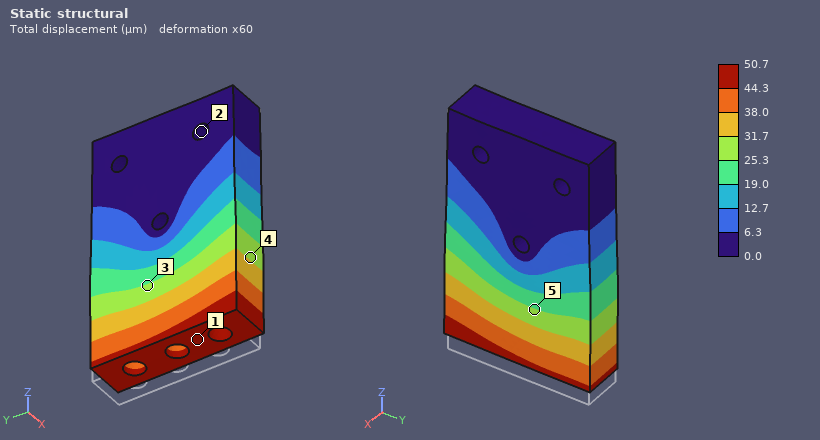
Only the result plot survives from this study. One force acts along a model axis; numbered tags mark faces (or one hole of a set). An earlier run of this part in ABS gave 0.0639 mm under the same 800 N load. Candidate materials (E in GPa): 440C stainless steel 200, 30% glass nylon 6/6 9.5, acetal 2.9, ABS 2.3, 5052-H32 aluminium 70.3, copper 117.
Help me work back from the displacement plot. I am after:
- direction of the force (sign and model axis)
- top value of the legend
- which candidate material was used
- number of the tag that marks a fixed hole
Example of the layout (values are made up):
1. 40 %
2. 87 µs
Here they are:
1. +Z
2. 50.7 µm
3. acetal
4. 2
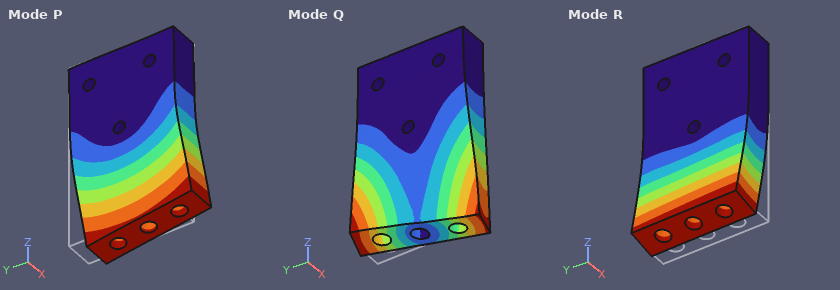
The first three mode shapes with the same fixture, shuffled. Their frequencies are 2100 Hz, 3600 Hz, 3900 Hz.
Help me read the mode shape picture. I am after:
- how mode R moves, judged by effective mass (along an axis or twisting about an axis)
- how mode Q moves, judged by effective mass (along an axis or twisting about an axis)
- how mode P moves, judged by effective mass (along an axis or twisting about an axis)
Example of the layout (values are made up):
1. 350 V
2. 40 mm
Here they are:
1. along X
2. twisting about Z
3. along Y
